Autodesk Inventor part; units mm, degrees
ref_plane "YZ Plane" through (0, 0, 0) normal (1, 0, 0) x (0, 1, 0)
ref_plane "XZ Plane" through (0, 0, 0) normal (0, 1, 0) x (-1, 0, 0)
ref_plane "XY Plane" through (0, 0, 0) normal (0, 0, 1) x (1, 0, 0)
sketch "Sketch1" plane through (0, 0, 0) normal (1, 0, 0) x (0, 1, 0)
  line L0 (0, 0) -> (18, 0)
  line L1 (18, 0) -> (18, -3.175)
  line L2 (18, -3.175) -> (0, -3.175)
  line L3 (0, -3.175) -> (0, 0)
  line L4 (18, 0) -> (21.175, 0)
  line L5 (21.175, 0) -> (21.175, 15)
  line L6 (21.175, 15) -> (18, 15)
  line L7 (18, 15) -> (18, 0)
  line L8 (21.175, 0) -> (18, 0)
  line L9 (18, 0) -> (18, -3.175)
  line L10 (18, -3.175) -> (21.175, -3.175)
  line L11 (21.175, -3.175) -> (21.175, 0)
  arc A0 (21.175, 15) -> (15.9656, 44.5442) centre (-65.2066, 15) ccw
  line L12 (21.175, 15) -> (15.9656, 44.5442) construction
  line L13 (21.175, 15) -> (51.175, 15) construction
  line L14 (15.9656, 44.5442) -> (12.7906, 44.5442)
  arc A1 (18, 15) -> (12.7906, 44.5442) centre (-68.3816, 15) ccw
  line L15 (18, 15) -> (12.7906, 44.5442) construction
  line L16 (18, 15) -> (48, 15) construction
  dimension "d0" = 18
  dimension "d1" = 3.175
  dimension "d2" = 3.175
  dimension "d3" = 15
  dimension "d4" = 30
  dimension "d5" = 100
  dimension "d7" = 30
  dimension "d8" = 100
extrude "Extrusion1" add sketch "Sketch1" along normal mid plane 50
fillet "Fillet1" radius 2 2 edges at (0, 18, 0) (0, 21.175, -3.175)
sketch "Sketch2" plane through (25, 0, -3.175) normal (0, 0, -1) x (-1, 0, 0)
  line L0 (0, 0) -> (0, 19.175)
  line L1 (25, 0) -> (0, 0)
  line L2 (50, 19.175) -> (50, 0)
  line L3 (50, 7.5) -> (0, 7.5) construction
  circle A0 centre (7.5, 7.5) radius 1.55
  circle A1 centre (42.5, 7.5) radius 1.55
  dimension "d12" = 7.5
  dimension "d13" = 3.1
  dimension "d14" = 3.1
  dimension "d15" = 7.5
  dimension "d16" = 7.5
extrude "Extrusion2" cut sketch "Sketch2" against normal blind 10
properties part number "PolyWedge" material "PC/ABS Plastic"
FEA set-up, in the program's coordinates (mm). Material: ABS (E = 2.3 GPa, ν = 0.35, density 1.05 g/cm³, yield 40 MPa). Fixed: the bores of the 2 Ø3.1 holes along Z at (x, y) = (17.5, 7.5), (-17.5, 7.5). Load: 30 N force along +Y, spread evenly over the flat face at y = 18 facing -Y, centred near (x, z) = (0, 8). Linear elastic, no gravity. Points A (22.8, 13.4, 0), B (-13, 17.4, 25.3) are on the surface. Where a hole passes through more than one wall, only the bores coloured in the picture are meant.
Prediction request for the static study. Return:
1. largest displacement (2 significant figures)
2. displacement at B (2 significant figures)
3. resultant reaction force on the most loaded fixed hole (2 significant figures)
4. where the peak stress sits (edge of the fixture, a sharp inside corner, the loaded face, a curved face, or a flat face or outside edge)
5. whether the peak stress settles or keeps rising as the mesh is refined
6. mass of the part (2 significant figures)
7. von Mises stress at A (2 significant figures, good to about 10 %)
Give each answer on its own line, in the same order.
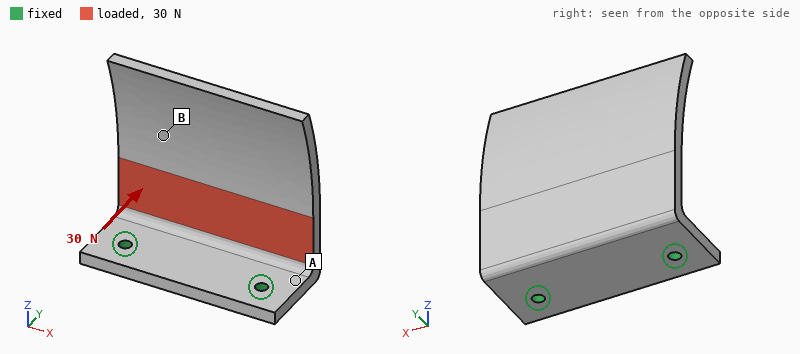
0.71 mm
0.41 mm
15 N
edge of the fixture
keeps rising
11 g
3.9 MPa
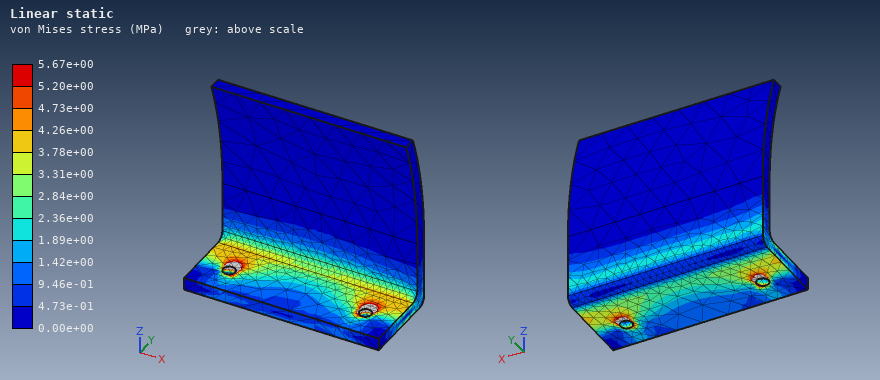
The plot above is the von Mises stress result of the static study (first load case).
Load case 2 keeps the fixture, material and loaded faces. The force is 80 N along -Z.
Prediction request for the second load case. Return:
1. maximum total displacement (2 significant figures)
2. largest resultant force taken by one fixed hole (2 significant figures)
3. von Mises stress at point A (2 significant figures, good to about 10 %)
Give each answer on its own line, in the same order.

0.73 mm
40 N
5.3 MPa
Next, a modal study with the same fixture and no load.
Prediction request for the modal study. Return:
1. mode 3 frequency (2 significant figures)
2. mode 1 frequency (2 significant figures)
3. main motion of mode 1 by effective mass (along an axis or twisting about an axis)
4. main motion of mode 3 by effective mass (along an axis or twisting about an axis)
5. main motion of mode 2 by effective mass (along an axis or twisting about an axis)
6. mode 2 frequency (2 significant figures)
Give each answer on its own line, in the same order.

1000 Hz
260 Hz
along Y
along X
along X
640 Hz
